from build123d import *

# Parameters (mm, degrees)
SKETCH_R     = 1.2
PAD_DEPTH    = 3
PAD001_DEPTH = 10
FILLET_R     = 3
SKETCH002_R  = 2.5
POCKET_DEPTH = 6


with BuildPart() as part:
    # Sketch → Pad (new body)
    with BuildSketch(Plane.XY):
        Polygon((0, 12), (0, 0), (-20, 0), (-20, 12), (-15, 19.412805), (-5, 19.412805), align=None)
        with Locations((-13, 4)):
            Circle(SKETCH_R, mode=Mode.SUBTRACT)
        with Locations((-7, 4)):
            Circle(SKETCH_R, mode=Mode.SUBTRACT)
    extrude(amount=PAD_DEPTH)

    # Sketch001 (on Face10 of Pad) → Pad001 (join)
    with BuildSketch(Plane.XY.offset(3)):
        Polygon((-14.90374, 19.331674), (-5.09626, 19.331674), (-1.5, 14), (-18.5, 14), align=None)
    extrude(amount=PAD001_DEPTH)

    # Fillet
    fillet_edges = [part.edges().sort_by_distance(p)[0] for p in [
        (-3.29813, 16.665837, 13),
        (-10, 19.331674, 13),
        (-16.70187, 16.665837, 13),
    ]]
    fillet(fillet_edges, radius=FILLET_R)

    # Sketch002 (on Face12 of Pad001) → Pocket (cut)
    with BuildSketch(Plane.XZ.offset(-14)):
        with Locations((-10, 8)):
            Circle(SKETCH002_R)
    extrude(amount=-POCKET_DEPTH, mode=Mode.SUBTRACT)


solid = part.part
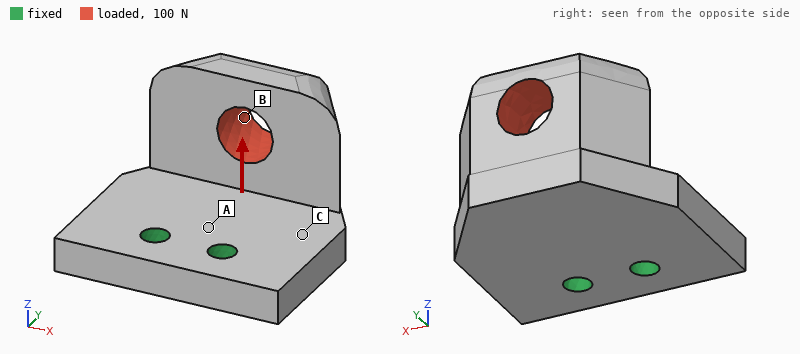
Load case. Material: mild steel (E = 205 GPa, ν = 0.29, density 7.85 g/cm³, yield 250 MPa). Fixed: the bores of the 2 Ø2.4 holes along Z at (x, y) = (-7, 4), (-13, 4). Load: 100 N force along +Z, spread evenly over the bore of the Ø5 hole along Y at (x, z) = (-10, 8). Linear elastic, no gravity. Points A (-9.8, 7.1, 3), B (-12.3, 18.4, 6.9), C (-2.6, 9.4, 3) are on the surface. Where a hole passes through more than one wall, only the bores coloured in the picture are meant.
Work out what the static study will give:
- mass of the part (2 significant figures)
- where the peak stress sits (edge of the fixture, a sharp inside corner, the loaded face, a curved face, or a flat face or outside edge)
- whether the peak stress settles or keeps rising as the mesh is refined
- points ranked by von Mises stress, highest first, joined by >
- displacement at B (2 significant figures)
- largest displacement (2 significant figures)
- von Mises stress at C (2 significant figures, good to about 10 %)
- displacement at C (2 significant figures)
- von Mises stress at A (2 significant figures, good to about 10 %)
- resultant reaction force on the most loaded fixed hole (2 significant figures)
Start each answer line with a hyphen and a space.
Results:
- 13 g
- edge of the fixture
- keeps rising
- A > C > B
- 11 µm
- 13 µm
- 21 MPa
- 2.1 µm
- 32 MPa
- 50 N
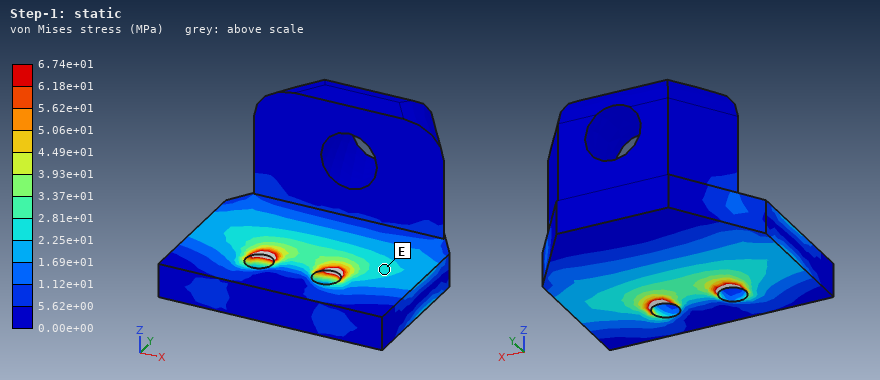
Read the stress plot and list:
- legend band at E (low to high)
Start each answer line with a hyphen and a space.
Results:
- 2.25e+01 to 2.81e+01 MPa
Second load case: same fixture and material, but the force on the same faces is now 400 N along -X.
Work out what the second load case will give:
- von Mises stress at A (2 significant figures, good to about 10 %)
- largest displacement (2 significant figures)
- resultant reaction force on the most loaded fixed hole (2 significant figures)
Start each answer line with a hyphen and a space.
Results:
- 84 MPa
- 21 µm
- 660 N
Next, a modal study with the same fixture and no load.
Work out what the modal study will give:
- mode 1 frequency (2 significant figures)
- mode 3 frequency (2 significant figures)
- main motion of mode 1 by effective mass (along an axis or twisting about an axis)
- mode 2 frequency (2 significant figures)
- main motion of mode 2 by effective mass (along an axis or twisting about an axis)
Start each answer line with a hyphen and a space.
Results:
- 5800 Hz
- 19 kHz
- along Z
- 11 kHz
- along X
